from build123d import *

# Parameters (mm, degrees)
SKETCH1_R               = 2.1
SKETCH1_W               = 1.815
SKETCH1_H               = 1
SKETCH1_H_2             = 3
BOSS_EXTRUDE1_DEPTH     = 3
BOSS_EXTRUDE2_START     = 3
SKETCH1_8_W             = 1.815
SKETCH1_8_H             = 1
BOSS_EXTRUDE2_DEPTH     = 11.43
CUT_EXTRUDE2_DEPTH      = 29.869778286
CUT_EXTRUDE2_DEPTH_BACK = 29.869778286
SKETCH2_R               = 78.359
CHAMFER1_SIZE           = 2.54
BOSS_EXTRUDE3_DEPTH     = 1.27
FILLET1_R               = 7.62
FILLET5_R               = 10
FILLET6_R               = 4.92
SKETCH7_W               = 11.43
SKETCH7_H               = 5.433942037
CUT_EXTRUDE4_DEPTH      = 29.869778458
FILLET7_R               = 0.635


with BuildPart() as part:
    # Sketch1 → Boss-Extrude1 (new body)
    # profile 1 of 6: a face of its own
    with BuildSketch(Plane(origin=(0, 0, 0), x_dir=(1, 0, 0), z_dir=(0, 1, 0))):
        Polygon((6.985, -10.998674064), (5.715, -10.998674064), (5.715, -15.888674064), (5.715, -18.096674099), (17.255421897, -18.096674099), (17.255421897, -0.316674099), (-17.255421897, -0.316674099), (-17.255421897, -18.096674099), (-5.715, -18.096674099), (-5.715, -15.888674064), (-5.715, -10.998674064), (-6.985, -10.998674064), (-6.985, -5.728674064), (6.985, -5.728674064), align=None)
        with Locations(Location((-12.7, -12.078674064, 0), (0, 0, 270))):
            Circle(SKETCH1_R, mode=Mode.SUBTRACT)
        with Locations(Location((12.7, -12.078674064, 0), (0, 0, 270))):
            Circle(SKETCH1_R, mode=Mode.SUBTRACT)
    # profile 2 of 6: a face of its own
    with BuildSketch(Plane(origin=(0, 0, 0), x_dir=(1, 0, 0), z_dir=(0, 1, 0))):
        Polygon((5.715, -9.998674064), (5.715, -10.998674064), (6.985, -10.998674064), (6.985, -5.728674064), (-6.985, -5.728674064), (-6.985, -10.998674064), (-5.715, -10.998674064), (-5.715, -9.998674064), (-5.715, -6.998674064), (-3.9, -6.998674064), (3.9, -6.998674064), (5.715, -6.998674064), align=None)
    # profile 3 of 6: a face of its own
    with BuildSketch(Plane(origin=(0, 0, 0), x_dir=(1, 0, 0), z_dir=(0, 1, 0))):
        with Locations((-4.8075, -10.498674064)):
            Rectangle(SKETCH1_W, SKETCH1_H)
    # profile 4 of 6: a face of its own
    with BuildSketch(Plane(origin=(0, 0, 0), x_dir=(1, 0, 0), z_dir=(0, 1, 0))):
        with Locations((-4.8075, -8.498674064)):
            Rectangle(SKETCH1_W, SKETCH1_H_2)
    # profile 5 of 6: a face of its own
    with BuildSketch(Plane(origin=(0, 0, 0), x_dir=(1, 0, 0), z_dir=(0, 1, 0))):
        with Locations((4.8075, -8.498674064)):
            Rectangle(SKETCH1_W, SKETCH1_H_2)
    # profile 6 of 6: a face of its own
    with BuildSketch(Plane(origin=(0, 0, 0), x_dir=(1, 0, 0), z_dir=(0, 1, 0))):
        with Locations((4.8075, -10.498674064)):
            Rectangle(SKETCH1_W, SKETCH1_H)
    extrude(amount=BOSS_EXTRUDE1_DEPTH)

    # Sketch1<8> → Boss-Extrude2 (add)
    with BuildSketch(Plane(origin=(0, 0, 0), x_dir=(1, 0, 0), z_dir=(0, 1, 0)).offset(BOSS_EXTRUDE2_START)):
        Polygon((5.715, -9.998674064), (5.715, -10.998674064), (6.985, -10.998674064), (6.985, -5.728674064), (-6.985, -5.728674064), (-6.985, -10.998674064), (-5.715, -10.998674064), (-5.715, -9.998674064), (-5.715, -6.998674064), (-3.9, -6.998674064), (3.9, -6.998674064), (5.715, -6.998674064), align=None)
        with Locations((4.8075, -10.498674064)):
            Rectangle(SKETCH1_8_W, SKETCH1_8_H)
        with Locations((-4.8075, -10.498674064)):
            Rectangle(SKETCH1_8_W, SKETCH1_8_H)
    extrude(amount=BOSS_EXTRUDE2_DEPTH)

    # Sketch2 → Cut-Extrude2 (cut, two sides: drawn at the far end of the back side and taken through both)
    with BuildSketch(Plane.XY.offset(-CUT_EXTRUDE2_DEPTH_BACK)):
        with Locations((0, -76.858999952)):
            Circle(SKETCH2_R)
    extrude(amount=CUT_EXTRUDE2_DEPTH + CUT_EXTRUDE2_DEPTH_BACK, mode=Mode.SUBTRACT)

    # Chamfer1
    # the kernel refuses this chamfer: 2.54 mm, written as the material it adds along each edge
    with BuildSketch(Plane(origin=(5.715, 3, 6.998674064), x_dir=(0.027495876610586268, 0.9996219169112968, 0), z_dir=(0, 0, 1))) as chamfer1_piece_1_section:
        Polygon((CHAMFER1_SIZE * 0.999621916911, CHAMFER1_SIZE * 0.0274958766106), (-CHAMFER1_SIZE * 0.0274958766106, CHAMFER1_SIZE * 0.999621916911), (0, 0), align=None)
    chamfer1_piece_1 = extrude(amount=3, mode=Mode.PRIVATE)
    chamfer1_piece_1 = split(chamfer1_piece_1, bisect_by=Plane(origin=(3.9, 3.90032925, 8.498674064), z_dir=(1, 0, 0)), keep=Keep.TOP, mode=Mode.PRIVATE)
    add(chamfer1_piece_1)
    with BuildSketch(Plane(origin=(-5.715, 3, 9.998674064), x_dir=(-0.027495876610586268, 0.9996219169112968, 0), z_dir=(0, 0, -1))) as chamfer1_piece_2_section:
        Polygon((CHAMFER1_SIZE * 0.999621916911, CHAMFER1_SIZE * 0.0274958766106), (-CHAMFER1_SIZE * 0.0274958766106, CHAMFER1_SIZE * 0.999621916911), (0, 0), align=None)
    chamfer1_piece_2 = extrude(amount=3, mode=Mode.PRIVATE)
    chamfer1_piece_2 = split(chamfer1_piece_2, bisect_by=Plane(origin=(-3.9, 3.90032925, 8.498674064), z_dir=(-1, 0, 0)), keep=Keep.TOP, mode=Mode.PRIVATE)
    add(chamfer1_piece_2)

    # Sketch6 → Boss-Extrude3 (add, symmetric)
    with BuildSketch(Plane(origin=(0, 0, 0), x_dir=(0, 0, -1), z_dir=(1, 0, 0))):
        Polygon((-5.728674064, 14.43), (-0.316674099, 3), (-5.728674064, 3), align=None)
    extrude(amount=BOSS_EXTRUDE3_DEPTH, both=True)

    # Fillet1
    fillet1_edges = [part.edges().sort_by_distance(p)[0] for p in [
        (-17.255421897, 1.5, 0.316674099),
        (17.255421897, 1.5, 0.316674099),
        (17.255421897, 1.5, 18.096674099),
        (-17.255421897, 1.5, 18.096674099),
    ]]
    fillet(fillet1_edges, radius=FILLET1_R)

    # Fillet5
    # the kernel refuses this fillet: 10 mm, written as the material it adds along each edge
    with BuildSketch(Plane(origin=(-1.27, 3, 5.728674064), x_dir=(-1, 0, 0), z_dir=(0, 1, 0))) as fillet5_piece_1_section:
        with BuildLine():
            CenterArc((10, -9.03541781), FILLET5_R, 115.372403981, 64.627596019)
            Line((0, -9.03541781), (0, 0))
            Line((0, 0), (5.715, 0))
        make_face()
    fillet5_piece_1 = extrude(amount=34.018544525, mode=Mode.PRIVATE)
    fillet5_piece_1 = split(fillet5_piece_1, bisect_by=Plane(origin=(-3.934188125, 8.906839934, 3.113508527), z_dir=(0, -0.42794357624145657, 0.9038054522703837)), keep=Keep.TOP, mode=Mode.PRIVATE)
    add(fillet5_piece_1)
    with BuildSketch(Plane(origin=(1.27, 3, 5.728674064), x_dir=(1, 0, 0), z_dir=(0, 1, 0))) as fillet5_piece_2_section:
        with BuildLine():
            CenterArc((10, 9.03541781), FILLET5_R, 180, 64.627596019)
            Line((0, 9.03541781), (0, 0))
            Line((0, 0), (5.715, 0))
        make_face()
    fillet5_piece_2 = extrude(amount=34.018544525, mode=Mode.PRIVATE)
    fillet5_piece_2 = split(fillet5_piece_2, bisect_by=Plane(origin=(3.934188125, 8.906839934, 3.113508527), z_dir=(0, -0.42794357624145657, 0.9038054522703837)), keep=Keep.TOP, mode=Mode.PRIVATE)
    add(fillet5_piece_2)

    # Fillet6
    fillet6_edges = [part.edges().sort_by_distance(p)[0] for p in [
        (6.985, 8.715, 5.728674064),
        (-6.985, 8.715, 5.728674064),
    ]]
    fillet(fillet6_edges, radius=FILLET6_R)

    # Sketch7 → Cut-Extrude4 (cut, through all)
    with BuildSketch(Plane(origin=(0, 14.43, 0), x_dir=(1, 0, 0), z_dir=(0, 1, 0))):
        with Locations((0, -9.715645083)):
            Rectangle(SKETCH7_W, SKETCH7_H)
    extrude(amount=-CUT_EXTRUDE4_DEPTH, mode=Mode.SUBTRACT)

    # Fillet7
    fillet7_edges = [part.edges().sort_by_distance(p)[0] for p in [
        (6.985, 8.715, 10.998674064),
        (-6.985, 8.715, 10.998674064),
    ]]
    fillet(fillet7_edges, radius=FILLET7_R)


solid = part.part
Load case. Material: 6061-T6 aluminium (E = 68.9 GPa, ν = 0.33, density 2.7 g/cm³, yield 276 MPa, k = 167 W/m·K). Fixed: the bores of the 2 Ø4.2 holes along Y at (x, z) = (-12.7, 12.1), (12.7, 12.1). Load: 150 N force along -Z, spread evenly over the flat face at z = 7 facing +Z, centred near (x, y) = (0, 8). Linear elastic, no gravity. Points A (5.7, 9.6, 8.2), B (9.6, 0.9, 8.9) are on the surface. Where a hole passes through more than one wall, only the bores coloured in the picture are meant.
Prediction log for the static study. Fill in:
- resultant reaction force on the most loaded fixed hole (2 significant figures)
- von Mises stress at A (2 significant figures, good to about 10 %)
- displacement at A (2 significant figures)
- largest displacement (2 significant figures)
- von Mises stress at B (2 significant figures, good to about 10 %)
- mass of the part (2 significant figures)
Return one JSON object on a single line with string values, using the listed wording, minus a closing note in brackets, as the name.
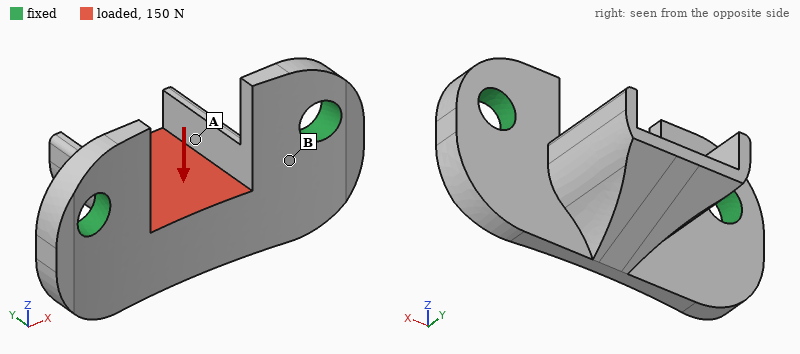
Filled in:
{"resultant reaction force on the most loaded fixed hole": "76 N", "von Mises stress at A": "11 MPa", "displacement at A": "27 µm", "largest displacement": "48 µm", "von Mises stress at B": "31 MPa", "mass of the part": "3.9 g"}
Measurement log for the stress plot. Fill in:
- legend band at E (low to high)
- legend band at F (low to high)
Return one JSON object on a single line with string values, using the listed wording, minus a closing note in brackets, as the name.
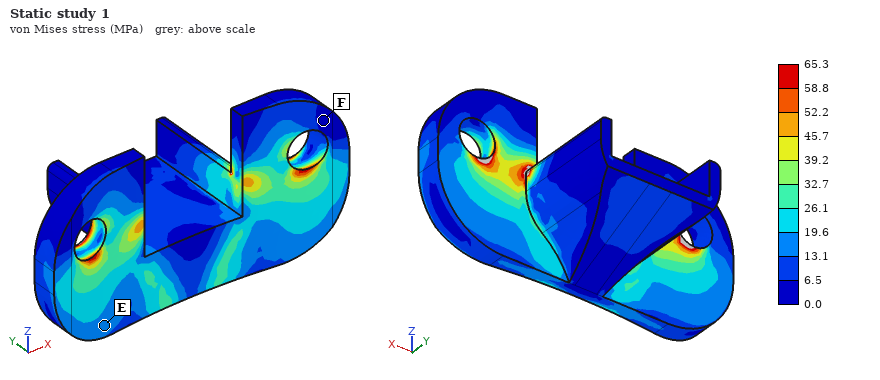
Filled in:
{"legend band at E": "13.1 to 19.6 MPa", "legend band at F": "0.0 to 6.5 MPa"}
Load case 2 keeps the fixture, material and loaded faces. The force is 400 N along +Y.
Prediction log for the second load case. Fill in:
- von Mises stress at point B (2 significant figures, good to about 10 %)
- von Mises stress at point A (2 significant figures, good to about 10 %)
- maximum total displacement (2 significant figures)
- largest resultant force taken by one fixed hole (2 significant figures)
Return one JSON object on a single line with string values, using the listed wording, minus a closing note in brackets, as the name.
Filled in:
{"von Mises stress at point B": "67 MPa", "von Mises stress at point A": "16 MPa", "maximum total displacement": "53 µm", "largest resultant force taken by one fixed hole": "220 N"}
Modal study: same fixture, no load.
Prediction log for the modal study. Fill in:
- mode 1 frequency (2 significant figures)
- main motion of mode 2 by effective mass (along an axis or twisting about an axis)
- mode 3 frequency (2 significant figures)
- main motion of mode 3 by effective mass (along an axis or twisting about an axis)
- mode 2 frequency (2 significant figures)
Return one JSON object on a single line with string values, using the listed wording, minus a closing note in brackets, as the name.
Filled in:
{"mode 1 frequency": "7200 Hz", "main motion of mode 2 by effective mass": "along X", "mode 3 frequency": "20 kHz", "main motion of mode 3 by effective mass": "along Y", "mode 2 frequency": "17 kHz"}
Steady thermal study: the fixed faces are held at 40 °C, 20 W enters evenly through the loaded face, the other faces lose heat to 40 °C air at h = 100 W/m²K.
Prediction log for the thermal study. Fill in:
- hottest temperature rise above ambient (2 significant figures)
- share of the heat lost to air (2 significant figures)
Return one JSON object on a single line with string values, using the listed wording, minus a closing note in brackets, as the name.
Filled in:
{"hottest temperature rise above ambient": "37 K", "share of the heat lost to air": "11 %"}
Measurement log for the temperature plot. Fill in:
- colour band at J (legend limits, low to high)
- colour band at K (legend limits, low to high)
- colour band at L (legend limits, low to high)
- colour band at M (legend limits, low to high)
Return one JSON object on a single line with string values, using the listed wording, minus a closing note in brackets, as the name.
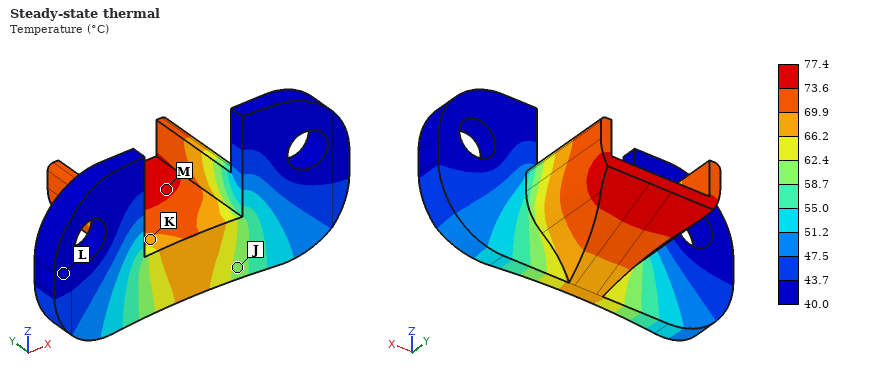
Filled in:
{"colour band at J": "58.7 to 62.4 °C", "colour band at K": "66.2 to 69.9 °C", "colour band at L": "40.0 to 43.7 °C", "colour band at M": "73.6 to 77.4 °C"}
